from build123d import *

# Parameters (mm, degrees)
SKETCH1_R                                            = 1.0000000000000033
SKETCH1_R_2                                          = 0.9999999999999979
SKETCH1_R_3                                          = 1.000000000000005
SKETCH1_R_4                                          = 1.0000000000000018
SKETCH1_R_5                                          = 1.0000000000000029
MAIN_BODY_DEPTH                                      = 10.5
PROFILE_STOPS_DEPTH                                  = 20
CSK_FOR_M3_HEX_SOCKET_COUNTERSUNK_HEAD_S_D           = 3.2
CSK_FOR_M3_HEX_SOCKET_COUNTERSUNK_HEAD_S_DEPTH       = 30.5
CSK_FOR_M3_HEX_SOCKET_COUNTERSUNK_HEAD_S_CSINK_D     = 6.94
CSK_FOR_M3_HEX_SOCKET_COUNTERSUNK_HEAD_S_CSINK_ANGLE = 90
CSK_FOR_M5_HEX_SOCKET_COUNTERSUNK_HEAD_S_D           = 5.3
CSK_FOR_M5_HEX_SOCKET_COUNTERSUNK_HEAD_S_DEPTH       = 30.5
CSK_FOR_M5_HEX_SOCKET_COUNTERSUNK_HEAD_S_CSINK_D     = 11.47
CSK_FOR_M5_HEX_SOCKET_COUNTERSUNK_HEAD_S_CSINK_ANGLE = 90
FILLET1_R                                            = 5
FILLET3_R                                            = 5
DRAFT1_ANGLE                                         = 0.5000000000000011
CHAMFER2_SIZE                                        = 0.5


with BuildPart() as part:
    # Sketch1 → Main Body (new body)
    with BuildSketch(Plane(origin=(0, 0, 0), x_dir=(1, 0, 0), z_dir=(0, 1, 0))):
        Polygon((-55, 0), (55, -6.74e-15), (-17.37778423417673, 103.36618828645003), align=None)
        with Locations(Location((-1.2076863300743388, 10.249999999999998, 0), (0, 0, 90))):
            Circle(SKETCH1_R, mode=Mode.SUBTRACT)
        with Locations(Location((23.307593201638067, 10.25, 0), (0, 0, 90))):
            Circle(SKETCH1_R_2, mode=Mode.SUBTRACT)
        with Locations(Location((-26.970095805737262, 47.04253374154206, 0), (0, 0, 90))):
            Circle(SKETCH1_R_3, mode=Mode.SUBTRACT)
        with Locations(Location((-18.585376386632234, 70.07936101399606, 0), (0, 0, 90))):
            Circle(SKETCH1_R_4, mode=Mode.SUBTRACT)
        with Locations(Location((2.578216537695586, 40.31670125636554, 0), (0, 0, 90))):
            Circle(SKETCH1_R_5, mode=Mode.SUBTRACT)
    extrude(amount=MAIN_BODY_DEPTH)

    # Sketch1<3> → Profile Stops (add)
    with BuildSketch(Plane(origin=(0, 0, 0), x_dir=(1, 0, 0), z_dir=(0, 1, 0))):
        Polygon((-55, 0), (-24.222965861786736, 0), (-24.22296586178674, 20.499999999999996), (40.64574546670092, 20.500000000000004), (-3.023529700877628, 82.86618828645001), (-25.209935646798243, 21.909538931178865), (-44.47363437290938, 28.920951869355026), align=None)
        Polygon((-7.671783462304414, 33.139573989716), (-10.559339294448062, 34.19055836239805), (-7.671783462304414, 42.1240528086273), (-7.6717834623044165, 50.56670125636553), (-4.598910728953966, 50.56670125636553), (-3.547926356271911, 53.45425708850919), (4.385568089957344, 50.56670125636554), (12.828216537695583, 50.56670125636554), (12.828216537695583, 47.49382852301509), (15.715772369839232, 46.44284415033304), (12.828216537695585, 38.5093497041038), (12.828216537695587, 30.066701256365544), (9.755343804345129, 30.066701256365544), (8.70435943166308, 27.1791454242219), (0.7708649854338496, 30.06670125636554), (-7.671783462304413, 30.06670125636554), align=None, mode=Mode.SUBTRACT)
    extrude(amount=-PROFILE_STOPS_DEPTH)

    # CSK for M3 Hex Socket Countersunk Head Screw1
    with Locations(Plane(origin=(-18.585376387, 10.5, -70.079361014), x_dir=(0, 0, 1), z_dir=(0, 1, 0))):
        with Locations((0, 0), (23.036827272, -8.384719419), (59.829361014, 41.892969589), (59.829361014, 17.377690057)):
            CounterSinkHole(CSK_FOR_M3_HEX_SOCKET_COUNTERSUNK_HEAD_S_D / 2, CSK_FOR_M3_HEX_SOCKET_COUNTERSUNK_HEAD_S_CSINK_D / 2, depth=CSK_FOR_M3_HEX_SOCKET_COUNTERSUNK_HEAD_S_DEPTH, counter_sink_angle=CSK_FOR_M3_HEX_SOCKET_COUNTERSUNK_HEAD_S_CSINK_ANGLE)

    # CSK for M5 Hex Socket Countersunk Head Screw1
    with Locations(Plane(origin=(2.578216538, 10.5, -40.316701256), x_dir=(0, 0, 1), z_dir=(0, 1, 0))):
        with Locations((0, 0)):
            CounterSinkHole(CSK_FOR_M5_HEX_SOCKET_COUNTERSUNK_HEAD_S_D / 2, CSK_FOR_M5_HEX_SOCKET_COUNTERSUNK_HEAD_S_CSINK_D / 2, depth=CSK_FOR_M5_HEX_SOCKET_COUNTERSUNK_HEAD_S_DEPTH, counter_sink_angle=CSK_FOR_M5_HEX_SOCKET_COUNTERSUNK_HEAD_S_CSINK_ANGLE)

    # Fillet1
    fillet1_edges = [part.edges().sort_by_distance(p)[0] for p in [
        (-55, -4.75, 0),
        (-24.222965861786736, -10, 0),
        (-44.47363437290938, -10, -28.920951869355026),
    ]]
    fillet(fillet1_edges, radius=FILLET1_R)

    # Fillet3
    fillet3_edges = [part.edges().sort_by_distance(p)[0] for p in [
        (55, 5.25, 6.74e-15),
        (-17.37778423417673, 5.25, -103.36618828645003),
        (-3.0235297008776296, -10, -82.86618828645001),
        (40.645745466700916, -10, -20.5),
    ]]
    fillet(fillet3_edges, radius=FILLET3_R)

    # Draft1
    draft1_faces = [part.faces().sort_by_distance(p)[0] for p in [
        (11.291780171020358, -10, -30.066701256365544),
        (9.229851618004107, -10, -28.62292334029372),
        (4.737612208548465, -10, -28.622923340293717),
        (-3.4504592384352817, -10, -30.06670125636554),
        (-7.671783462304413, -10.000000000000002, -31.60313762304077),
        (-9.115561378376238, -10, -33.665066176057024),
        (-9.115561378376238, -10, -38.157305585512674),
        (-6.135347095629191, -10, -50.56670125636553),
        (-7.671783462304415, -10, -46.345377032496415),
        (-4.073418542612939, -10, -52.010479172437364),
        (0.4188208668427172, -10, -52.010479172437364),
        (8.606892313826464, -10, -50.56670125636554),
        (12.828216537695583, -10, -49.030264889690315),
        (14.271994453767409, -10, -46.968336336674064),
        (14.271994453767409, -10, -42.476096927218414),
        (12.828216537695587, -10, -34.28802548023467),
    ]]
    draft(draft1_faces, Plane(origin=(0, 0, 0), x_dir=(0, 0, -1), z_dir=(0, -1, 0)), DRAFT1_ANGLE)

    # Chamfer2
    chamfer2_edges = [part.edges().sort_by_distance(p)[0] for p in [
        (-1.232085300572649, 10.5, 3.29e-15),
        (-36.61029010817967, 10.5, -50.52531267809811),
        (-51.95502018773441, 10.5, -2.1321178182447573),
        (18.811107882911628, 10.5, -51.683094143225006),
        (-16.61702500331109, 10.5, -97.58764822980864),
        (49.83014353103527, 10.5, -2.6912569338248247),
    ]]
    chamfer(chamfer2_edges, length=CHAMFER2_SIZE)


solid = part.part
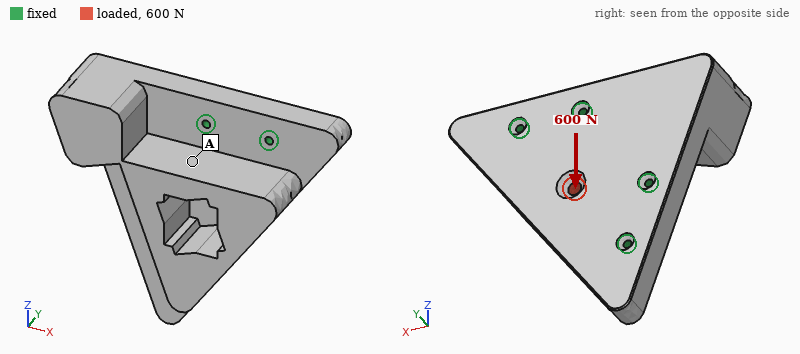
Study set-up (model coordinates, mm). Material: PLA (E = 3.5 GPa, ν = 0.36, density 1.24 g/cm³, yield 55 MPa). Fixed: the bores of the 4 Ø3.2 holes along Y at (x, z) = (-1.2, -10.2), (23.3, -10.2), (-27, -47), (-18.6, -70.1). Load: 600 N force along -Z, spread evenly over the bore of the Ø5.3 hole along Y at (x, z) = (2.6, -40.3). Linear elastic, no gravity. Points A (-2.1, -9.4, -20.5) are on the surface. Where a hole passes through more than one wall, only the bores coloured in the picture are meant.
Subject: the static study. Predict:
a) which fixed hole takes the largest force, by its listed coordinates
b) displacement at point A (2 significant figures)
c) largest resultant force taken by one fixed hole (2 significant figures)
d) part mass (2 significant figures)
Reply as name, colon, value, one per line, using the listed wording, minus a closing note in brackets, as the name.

which fixed hole takes the largest force, by its listed coordinates: (-1.2, -10.2)
displacement at point A: 7.4 µm
largest resultant force taken by one fixed hole: 220 N
part mass: 130 g
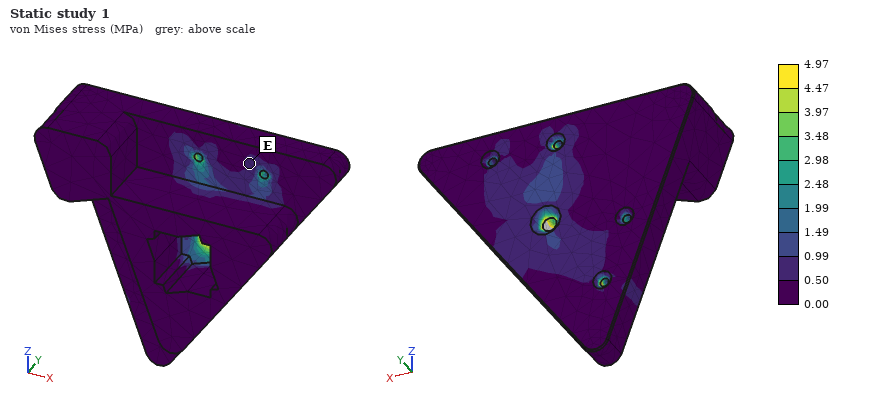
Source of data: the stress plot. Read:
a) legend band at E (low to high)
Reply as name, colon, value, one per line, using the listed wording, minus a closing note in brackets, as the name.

legend band at E: 0.50 to 0.99 MPa
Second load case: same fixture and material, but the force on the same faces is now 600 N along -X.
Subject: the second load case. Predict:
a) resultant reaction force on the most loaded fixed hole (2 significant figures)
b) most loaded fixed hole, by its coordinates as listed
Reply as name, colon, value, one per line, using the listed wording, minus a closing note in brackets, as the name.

resultant reaction force on the most loaded fixed hole: 250 N
most loaded fixed hole, by its coordinates as listed: (-27, -47)
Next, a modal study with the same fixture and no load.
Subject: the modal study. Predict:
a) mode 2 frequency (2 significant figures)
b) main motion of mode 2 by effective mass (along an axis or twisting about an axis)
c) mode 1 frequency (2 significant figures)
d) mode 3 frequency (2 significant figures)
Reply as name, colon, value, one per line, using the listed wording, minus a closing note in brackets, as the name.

mode 2 frequency: 2200 Hz
main motion of mode 2 by effective mass: along Y
mode 1 frequency: 1300 Hz
mode 3 frequency: 2900 Hz
